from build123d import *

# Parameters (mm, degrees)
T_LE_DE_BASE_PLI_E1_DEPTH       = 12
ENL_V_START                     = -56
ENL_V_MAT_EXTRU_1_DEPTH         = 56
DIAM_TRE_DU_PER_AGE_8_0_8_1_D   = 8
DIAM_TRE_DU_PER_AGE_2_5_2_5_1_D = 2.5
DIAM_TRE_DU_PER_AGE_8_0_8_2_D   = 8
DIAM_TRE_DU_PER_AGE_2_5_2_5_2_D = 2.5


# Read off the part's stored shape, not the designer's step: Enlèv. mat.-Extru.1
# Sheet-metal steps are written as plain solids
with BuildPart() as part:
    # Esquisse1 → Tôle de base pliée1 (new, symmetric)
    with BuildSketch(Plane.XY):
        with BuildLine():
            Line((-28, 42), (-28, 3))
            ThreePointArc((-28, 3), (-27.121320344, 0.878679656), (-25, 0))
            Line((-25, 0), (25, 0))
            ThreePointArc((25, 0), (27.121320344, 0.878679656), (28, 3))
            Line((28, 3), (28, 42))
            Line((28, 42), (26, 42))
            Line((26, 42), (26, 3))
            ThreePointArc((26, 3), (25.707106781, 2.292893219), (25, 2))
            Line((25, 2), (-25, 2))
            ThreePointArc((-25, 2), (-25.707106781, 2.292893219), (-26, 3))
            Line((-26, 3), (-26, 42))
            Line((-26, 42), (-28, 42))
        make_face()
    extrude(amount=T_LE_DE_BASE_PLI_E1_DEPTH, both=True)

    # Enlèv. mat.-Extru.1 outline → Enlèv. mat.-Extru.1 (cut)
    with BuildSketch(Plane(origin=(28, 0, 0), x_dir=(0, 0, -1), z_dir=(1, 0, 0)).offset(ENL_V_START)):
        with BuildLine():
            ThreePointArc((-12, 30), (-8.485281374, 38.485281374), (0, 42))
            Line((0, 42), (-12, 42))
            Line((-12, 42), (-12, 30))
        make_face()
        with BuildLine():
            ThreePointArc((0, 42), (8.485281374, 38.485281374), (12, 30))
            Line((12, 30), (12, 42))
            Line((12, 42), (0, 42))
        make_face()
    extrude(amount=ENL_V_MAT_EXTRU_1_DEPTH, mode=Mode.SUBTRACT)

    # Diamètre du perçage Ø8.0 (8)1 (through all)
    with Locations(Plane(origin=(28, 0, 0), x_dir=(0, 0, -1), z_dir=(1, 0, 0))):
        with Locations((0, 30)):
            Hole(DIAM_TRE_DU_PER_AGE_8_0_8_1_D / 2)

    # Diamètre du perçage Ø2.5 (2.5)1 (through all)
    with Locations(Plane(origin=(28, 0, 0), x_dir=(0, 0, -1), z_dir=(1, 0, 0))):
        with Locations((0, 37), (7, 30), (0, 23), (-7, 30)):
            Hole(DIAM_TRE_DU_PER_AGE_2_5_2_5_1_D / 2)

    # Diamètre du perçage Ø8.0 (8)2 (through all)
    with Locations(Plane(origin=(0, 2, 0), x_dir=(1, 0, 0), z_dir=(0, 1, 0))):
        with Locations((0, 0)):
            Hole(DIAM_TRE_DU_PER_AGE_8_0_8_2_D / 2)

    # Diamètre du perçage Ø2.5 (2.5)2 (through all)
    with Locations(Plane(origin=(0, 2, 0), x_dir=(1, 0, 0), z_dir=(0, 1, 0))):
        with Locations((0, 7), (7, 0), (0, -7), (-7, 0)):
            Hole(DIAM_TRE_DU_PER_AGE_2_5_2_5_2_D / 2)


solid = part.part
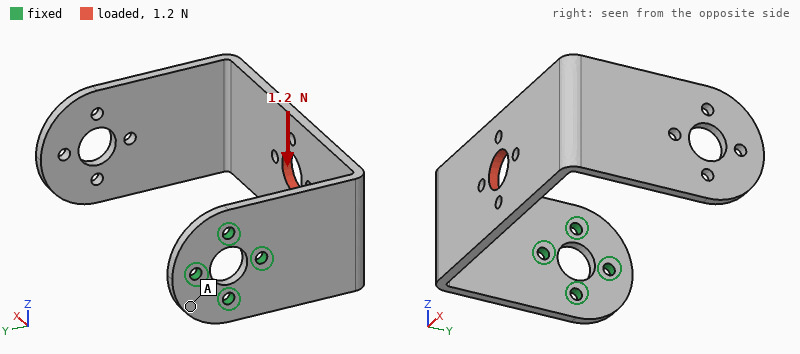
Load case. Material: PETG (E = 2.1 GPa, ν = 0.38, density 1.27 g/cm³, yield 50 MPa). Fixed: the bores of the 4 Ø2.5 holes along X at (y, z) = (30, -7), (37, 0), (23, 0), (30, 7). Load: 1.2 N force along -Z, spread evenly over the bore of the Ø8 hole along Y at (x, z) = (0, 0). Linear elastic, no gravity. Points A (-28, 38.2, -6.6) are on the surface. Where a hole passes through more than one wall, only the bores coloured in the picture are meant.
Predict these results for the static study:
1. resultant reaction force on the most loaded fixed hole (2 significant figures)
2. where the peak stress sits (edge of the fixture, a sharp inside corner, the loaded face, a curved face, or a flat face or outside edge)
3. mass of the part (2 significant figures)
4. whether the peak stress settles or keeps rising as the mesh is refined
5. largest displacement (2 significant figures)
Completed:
1.5 N
edge of the fixture
7.3 g
keeps rising
0.81 mm
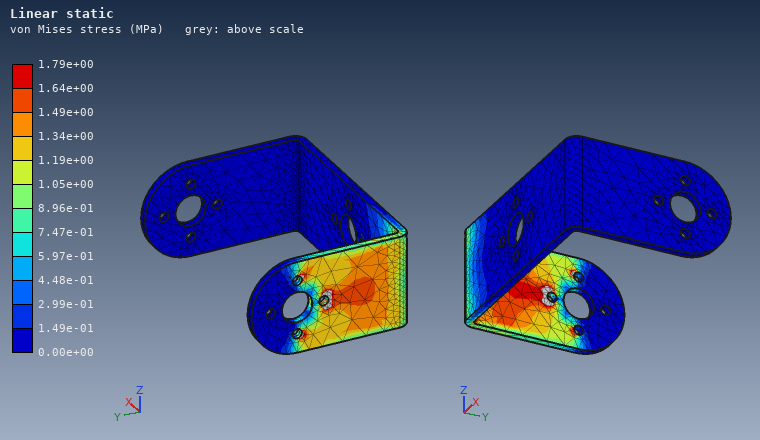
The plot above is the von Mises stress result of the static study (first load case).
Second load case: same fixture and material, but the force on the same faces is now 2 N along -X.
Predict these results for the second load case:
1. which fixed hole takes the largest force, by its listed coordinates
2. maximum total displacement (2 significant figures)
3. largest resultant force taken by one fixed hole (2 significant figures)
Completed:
(23, 0)
0.84 mm
4.7 N
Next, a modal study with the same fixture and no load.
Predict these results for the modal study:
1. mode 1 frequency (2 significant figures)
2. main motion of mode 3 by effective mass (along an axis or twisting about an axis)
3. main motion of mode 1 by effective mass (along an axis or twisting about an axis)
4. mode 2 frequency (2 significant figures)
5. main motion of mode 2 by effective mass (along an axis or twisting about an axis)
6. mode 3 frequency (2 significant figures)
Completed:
47 Hz
along X
along Y
72 Hz
along Z
150 Hz
